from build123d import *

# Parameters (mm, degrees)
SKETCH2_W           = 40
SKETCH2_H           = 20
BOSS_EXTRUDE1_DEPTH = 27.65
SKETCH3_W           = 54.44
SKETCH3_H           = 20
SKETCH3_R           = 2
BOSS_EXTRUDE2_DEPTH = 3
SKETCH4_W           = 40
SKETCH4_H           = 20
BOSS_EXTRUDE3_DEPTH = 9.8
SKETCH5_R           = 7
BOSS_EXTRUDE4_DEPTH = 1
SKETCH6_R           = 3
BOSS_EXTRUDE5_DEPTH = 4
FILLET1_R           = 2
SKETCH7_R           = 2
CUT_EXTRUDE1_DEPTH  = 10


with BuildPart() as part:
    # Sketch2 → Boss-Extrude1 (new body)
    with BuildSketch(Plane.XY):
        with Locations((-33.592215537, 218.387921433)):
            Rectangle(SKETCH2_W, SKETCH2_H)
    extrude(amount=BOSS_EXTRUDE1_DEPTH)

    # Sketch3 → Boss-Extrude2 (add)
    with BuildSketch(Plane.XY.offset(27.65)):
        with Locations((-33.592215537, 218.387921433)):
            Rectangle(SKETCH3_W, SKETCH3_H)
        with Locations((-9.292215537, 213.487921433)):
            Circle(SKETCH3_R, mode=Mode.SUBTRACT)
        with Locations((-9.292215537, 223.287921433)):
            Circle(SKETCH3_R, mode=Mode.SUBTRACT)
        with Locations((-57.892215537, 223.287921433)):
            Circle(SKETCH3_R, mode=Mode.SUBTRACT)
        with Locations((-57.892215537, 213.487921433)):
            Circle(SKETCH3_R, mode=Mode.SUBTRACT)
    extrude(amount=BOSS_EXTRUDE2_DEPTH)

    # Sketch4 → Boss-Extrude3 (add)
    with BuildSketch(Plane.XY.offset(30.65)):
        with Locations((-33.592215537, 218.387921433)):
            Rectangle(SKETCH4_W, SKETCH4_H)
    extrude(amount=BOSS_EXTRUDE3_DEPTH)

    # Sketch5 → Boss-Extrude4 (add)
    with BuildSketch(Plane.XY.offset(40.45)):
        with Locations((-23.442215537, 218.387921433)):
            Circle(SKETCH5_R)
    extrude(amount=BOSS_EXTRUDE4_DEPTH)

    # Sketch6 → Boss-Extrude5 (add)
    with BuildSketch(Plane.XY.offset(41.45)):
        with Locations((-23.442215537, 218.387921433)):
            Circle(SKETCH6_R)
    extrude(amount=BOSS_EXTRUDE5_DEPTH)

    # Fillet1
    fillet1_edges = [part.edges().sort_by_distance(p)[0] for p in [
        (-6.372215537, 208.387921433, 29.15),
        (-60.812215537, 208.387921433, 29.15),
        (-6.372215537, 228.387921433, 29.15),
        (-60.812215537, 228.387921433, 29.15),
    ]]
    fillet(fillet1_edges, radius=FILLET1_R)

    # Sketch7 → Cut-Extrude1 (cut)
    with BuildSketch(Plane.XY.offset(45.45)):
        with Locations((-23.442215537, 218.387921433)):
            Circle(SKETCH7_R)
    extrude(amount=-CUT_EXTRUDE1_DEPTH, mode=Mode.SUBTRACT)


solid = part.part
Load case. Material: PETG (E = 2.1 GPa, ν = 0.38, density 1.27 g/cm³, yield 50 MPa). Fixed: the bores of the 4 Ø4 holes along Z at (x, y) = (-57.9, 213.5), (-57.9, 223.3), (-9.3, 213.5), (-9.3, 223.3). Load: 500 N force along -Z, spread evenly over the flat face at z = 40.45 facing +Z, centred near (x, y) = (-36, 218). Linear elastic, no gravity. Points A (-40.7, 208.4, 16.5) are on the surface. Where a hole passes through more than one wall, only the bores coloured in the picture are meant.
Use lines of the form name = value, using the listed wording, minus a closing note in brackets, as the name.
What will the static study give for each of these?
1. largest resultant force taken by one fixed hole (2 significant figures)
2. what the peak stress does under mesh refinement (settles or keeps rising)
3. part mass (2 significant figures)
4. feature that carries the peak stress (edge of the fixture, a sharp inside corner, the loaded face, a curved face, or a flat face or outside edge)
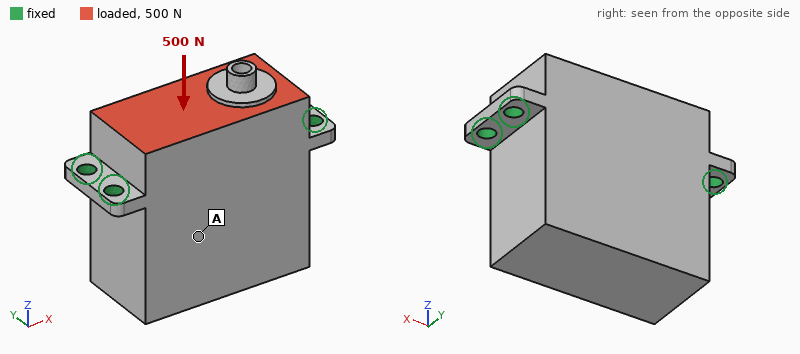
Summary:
largest resultant force taken by one fixed hole = 140 N
what the peak stress does under mesh refinement = keeps rising
part mass = 42 g
feature that carries the peak stress = edge of the fixture
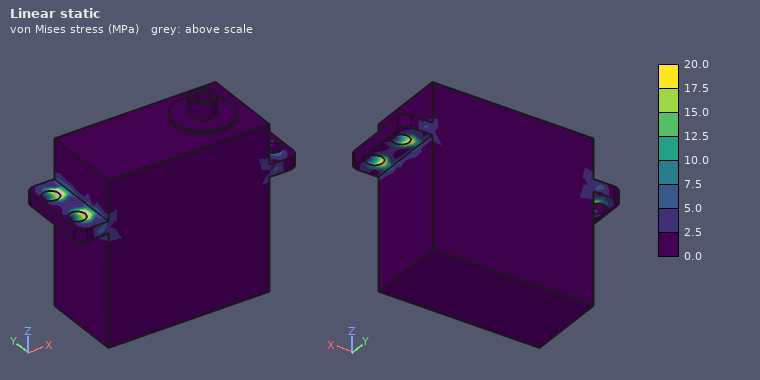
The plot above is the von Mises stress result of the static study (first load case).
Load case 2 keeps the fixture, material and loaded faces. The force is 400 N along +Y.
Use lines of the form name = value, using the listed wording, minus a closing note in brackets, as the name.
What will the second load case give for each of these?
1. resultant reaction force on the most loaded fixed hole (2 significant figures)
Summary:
resultant reaction force on the most loaded fixed hole = 220 N
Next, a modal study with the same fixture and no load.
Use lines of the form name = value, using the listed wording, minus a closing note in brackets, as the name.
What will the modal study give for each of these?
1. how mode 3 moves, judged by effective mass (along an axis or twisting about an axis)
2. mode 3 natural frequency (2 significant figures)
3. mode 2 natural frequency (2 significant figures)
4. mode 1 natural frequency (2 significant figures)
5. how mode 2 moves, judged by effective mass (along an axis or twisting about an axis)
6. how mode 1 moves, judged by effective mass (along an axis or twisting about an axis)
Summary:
how mode 3 moves, judged by effective mass = along X
mode 3 natural frequency = 2700 Hz
mode 2 natural frequency = 2500 Hz
mode 1 natural frequency = 920 Hz
how mode 2 moves, judged by effective mass = along Z
how mode 1 moves, judged by effective mass = along Y
